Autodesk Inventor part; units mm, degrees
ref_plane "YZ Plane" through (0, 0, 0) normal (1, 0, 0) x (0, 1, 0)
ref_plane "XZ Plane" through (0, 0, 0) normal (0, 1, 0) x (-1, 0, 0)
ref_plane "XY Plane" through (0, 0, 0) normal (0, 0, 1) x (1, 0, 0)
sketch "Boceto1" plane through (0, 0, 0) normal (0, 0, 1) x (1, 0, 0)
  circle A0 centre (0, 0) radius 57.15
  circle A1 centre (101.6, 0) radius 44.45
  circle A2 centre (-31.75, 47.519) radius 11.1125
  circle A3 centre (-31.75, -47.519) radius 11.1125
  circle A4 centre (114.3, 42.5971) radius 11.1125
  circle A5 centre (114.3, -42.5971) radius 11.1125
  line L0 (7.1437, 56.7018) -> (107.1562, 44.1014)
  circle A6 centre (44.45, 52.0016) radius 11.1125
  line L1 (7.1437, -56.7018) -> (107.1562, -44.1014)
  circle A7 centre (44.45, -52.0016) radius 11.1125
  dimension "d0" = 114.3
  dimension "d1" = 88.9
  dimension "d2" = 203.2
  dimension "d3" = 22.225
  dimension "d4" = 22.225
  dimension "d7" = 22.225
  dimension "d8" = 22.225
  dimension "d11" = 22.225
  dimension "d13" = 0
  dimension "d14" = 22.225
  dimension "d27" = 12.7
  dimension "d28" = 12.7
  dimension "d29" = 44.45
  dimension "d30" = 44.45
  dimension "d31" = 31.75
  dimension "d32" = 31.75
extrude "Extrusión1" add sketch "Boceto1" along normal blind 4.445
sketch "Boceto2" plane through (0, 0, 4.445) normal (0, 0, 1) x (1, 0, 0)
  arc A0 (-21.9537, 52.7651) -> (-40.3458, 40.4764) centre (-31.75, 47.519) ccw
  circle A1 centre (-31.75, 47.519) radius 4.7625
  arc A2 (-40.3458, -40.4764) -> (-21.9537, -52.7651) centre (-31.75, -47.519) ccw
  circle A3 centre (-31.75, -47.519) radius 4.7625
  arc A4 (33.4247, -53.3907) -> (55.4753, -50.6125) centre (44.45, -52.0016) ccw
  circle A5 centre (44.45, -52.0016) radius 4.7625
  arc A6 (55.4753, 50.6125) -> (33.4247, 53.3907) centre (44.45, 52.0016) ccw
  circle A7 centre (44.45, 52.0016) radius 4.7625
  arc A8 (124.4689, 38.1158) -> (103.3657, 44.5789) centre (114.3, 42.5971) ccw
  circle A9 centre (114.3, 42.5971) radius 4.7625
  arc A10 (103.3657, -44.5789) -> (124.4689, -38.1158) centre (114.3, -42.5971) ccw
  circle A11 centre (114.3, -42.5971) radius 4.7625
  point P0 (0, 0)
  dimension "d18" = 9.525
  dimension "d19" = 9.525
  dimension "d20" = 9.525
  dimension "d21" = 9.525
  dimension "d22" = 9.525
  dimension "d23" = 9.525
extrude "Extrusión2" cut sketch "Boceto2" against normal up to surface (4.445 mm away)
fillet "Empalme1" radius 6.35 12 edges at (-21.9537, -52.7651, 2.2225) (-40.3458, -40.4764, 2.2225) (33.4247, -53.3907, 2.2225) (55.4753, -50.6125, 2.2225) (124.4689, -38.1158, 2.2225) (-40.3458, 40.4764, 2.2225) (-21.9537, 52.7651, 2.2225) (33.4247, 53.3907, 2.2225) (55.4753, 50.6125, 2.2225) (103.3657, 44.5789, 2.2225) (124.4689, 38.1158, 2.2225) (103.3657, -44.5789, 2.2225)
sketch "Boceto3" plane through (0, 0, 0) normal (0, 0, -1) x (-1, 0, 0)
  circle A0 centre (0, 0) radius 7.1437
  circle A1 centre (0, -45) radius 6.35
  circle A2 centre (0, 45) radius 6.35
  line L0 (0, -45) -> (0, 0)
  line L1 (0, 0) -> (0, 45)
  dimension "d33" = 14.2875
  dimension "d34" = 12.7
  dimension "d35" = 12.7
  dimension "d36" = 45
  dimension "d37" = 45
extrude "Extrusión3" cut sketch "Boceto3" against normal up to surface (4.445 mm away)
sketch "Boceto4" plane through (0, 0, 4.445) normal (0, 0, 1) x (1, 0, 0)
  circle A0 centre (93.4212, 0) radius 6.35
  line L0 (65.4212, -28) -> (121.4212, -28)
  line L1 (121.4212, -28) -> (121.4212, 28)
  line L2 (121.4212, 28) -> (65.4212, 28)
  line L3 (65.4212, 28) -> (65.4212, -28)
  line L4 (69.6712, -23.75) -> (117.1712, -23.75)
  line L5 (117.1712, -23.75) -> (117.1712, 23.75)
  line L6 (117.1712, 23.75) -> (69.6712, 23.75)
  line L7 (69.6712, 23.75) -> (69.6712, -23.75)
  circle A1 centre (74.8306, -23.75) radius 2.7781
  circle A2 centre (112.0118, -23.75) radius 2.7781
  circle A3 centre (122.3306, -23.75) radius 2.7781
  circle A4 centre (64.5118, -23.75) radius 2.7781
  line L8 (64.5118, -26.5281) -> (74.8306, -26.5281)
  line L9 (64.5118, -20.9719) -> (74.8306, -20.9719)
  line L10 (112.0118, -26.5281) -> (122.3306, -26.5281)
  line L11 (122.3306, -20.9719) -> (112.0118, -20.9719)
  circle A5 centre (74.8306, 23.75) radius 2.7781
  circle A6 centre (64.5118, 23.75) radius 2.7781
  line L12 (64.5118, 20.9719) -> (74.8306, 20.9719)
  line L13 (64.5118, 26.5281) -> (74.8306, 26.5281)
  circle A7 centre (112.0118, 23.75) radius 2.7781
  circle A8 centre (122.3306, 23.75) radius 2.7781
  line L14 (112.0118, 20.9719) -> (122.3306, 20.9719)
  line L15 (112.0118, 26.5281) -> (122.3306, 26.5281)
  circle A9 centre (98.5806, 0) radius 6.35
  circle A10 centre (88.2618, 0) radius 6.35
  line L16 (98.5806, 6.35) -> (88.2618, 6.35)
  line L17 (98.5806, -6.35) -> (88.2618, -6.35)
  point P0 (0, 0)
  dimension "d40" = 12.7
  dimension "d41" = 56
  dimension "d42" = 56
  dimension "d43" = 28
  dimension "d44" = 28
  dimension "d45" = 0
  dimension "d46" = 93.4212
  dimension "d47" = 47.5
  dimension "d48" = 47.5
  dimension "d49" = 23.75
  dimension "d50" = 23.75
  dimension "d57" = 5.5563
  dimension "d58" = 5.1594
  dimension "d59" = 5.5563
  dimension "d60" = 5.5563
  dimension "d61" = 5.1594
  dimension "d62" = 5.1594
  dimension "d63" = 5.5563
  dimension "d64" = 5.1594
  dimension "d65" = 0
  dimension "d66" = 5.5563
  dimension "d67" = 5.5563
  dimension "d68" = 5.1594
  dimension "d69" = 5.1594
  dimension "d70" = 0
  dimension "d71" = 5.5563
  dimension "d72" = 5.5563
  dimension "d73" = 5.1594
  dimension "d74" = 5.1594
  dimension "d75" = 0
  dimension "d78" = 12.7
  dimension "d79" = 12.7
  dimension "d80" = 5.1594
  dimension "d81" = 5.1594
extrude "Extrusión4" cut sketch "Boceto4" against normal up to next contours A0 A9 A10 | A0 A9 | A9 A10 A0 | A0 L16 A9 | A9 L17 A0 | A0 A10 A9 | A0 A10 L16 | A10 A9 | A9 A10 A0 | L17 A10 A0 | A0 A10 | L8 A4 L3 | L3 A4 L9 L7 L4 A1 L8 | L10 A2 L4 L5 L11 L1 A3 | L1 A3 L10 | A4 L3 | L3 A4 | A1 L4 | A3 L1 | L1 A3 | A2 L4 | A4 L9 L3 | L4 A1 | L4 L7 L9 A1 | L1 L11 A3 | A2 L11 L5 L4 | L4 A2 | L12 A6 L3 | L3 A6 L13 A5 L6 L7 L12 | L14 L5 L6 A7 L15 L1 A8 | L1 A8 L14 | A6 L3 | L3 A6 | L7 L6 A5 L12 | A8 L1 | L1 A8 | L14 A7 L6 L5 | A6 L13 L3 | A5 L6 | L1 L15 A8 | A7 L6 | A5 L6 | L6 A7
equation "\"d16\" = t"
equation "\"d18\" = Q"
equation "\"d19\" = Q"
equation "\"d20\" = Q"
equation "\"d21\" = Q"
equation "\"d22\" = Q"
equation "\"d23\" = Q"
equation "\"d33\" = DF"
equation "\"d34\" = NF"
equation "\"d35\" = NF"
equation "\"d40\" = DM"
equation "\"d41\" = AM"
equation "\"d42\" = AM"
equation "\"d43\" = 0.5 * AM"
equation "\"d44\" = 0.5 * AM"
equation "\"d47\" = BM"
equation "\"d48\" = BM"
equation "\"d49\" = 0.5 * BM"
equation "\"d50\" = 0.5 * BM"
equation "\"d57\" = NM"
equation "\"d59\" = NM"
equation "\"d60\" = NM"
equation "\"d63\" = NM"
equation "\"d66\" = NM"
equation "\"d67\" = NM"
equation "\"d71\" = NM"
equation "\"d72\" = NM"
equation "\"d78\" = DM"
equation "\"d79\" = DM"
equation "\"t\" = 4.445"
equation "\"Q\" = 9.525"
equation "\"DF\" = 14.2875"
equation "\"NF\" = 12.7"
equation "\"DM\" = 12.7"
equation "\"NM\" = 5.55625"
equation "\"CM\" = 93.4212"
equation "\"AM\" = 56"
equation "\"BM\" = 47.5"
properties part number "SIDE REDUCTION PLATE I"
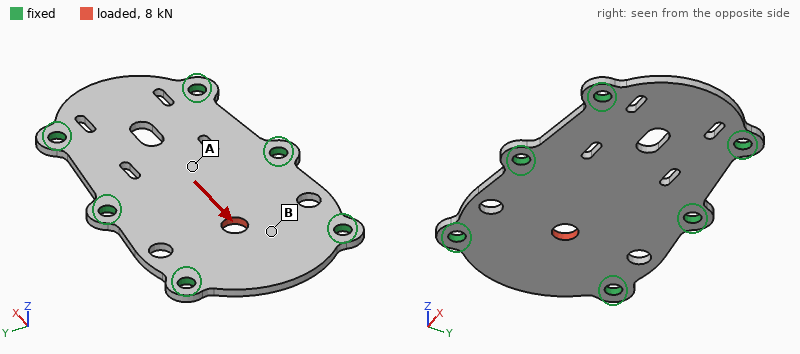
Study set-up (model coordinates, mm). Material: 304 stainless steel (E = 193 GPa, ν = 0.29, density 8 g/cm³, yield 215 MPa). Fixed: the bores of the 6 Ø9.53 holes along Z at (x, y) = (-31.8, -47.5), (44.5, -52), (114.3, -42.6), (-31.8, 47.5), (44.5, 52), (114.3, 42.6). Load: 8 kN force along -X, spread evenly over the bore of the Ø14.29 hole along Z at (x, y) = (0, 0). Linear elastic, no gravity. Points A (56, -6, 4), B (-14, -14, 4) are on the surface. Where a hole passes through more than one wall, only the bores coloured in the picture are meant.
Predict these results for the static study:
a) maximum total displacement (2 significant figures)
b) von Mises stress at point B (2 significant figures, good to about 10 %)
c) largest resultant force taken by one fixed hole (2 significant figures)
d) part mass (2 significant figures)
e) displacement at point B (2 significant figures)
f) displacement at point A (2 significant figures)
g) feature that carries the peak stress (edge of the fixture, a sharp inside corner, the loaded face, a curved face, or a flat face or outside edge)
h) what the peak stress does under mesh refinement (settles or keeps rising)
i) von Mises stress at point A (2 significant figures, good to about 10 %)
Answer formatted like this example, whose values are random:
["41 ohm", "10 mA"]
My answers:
["8.2 µm", "20 MPa", "1.9 kN", "660 g", "5.2 µm", "2.6 µm", "a sharp inside corner", "keeps rising", "9.0 MPa"]
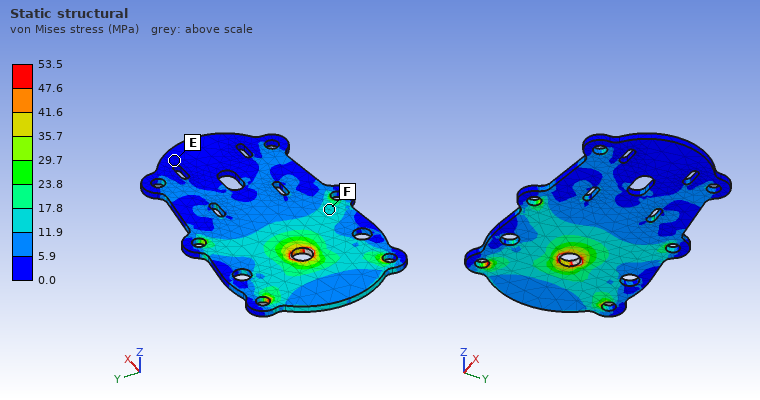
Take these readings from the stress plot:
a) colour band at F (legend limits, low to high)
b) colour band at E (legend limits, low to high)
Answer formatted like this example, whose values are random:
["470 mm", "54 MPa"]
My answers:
["11.9 to 17.8 MPa", "0.0 to 5.9 MPa"]
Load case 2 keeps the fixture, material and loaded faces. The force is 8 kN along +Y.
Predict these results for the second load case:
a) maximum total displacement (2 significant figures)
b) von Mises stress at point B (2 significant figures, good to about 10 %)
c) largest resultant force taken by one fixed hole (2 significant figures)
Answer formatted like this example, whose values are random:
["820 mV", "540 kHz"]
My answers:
["7.1 µm", "23 MPa", "2.4 kN"]
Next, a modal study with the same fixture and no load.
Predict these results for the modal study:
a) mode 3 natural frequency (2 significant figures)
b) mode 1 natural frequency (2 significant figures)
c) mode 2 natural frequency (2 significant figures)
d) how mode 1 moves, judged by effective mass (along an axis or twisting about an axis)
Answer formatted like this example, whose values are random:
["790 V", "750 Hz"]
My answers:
["2400 Hz", "2000 Hz", "2400 Hz", "along Z"]
